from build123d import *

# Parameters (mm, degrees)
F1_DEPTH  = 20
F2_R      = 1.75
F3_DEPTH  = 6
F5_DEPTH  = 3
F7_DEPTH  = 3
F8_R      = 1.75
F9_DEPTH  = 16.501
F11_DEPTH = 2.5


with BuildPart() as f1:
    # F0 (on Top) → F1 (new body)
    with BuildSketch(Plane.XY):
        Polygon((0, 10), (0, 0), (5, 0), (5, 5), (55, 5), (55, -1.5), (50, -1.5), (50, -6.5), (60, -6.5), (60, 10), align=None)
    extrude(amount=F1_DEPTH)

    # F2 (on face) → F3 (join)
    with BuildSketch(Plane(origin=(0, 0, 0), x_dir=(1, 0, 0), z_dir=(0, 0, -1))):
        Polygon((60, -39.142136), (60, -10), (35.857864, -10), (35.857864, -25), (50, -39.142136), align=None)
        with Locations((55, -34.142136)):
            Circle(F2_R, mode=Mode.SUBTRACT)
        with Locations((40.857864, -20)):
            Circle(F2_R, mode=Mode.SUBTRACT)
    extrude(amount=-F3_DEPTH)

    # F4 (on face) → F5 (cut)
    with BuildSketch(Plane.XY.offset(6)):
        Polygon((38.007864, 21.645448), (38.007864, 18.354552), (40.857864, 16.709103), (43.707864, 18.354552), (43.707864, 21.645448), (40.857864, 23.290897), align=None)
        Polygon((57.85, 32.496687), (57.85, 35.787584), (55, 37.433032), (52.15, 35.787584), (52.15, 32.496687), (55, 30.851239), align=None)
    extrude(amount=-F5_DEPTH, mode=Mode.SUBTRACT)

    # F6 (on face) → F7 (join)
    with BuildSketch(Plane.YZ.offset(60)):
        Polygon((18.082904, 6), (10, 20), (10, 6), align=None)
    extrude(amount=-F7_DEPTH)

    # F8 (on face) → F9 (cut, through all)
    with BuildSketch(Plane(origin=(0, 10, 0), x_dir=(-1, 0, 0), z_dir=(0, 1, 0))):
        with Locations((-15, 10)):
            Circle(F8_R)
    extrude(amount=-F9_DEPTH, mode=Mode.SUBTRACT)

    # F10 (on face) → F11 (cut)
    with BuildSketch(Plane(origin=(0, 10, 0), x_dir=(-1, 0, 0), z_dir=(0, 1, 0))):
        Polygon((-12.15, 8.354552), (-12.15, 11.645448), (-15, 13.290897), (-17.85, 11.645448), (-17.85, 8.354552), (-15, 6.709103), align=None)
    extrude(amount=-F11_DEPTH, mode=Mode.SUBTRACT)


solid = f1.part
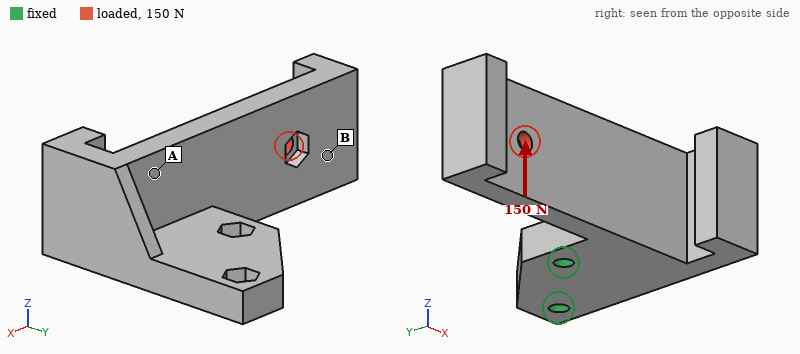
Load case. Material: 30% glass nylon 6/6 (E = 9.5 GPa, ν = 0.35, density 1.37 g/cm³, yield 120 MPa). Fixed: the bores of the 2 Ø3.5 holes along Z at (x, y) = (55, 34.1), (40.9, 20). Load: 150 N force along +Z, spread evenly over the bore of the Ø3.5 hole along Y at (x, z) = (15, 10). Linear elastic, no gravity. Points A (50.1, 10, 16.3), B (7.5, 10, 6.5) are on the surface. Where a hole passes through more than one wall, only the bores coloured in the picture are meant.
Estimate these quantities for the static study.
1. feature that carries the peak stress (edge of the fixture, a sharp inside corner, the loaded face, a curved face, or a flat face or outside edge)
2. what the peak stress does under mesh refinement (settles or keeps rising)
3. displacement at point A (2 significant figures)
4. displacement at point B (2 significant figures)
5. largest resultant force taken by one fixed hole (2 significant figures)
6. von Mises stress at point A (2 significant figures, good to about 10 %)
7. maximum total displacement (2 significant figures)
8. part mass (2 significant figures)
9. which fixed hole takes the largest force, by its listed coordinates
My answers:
edge of the fixture
keeps rising
0.17 mm
0.54 mm
350 N
11 MPa
0.75 mm
16 g
(40.9, 20)
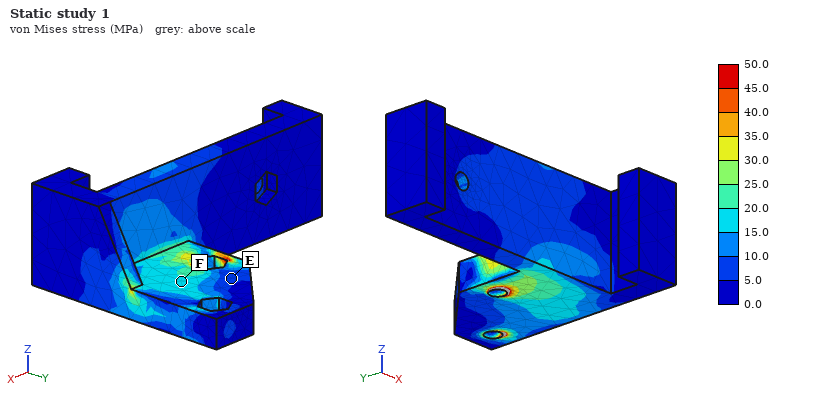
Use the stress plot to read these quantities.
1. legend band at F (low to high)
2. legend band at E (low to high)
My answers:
15.0 to 20.0 MPa
5.0 to 10.0 MPa
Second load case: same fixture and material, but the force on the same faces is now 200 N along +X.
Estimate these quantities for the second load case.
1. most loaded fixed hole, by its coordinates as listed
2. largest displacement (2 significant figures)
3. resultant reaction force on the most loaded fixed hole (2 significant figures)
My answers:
(40.9, 20)
0.26 mm
270 N
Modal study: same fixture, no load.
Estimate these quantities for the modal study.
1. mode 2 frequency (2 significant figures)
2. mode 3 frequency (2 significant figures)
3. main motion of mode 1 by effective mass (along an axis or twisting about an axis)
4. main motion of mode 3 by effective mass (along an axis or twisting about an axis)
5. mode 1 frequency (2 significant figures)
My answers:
1100 Hz
1600 Hz
along Y
along Z
920 Hz
